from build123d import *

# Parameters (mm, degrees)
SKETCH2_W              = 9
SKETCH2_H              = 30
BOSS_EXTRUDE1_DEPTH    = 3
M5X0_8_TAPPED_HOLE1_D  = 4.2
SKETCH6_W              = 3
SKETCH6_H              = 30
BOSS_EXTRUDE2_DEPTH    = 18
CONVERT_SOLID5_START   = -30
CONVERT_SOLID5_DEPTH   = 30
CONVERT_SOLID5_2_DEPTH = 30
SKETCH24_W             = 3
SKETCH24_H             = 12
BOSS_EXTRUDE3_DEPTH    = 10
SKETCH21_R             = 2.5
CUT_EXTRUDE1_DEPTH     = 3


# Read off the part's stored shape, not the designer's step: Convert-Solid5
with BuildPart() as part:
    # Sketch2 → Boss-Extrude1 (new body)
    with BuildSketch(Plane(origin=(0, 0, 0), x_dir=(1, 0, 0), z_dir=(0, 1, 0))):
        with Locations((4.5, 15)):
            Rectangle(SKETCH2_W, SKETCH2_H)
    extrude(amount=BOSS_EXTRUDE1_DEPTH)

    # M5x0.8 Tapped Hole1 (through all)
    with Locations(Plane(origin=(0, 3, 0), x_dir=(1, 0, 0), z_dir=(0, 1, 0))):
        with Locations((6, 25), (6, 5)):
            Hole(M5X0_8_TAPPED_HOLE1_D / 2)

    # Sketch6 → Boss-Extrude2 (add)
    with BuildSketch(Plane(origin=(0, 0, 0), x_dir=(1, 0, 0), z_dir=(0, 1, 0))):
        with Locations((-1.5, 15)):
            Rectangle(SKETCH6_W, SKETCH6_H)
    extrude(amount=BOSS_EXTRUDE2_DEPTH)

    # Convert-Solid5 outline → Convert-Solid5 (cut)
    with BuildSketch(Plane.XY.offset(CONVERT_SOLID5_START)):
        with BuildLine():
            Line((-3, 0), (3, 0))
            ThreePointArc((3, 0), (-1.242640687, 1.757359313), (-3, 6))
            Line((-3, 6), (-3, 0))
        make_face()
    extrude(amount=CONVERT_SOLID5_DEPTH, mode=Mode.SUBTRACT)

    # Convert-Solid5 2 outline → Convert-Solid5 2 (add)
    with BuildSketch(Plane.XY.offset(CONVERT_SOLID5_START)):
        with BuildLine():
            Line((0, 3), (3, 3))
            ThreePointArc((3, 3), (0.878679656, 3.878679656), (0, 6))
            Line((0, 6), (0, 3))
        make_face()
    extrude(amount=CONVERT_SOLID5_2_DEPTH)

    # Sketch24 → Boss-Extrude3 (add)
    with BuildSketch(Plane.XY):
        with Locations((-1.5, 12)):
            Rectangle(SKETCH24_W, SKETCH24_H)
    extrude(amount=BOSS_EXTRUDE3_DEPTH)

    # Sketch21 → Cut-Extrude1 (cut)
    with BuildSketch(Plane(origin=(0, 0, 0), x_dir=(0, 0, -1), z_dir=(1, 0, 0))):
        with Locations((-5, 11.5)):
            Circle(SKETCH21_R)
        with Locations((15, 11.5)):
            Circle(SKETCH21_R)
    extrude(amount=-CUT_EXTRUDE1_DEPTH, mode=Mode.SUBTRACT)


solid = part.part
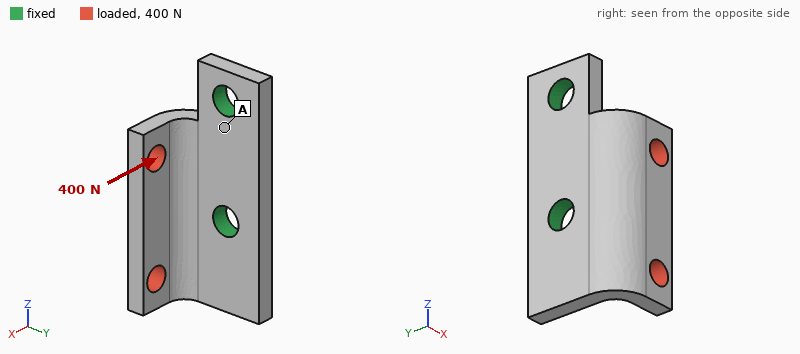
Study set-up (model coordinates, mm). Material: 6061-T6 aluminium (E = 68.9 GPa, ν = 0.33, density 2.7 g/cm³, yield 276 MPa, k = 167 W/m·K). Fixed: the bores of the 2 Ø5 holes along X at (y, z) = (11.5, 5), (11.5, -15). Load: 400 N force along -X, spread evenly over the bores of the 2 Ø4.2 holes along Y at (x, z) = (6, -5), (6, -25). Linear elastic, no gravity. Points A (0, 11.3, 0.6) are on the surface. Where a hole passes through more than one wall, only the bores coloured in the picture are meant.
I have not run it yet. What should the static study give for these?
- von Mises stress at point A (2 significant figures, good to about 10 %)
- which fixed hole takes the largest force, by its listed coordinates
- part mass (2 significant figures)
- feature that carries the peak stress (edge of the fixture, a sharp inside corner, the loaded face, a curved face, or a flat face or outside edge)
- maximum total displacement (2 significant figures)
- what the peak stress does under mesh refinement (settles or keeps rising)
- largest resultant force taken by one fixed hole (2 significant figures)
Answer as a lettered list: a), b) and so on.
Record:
a) 22 MPa
b) (11.5, -15)
c) 6.5 g
d) edge of the fixture
e) 68 µm
f) keeps rising
g) 370 N
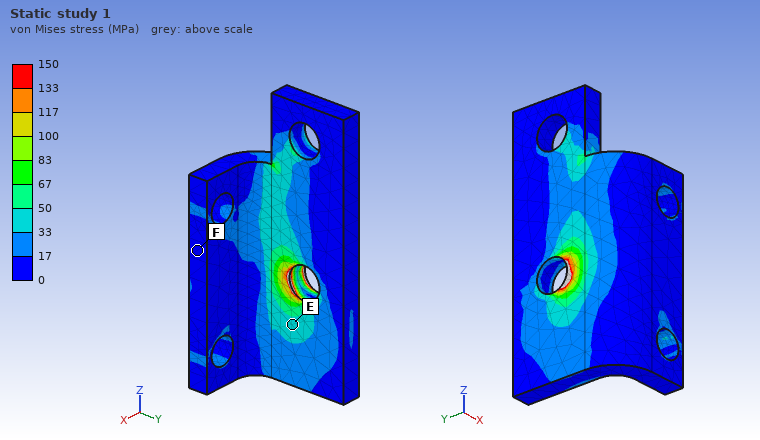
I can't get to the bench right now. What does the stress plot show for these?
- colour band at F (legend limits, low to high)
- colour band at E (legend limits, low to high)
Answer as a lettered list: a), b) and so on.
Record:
a) 0 to 17 MPa
b) 33 to 50 MPa
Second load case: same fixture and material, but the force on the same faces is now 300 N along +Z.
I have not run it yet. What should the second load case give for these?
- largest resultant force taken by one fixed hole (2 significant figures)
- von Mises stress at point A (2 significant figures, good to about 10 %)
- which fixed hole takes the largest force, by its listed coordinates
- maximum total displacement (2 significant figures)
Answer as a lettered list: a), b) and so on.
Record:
a) 250 N
b) 11 MPa
c) (11.5, -15)
d) 31 µm
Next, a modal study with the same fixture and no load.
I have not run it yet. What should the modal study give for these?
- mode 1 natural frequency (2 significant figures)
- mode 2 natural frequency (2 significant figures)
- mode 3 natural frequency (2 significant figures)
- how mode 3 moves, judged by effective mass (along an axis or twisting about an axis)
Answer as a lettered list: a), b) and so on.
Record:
a) 8700 Hz
b) 11 kHz
c) 17 kHz
d) along X
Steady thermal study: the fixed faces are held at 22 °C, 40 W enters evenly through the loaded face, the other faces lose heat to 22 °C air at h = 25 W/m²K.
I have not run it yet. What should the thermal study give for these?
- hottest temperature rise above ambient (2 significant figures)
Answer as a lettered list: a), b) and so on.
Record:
a) 61 K
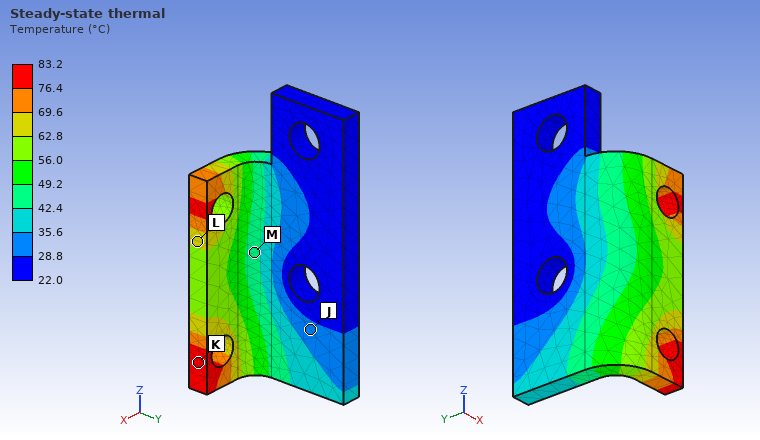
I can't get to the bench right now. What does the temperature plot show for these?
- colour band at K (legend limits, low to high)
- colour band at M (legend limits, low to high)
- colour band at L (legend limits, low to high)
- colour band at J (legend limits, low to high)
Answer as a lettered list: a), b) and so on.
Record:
a) 76.4 to 83.2 °C
b) 42.4 to 49.2 °C
c) 62.8 to 69.6 °C
d) 28.8 to 35.6 °C
